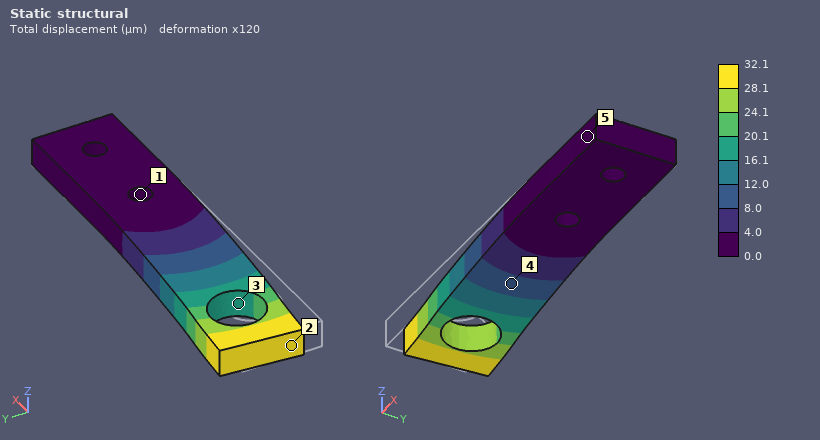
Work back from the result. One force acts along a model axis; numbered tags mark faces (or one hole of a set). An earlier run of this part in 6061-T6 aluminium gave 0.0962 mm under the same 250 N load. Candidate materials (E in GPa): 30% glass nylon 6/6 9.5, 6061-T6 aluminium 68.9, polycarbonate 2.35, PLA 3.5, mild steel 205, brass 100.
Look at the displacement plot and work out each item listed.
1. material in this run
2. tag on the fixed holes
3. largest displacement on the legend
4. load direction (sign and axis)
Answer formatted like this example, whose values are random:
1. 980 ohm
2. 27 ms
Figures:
1. mild steel
2. 1
3. 32.1 µm
4. +Y
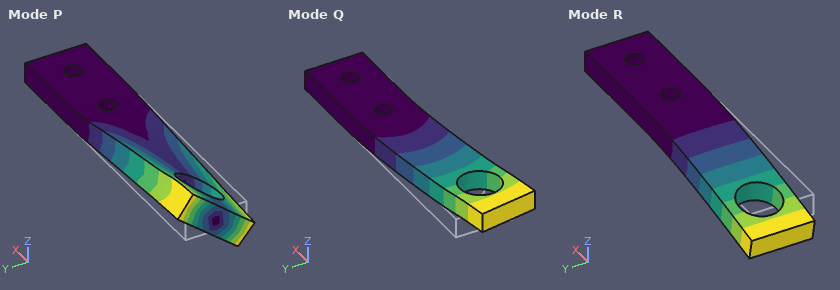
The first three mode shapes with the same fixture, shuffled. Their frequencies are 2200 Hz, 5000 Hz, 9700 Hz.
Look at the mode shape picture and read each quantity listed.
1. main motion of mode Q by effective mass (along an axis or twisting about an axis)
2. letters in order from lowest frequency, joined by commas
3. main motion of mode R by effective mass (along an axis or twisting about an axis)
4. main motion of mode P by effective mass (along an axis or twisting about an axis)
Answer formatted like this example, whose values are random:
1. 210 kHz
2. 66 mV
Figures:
1. along Y
2. R, Q, P
3. along Z
4. twisting about X
